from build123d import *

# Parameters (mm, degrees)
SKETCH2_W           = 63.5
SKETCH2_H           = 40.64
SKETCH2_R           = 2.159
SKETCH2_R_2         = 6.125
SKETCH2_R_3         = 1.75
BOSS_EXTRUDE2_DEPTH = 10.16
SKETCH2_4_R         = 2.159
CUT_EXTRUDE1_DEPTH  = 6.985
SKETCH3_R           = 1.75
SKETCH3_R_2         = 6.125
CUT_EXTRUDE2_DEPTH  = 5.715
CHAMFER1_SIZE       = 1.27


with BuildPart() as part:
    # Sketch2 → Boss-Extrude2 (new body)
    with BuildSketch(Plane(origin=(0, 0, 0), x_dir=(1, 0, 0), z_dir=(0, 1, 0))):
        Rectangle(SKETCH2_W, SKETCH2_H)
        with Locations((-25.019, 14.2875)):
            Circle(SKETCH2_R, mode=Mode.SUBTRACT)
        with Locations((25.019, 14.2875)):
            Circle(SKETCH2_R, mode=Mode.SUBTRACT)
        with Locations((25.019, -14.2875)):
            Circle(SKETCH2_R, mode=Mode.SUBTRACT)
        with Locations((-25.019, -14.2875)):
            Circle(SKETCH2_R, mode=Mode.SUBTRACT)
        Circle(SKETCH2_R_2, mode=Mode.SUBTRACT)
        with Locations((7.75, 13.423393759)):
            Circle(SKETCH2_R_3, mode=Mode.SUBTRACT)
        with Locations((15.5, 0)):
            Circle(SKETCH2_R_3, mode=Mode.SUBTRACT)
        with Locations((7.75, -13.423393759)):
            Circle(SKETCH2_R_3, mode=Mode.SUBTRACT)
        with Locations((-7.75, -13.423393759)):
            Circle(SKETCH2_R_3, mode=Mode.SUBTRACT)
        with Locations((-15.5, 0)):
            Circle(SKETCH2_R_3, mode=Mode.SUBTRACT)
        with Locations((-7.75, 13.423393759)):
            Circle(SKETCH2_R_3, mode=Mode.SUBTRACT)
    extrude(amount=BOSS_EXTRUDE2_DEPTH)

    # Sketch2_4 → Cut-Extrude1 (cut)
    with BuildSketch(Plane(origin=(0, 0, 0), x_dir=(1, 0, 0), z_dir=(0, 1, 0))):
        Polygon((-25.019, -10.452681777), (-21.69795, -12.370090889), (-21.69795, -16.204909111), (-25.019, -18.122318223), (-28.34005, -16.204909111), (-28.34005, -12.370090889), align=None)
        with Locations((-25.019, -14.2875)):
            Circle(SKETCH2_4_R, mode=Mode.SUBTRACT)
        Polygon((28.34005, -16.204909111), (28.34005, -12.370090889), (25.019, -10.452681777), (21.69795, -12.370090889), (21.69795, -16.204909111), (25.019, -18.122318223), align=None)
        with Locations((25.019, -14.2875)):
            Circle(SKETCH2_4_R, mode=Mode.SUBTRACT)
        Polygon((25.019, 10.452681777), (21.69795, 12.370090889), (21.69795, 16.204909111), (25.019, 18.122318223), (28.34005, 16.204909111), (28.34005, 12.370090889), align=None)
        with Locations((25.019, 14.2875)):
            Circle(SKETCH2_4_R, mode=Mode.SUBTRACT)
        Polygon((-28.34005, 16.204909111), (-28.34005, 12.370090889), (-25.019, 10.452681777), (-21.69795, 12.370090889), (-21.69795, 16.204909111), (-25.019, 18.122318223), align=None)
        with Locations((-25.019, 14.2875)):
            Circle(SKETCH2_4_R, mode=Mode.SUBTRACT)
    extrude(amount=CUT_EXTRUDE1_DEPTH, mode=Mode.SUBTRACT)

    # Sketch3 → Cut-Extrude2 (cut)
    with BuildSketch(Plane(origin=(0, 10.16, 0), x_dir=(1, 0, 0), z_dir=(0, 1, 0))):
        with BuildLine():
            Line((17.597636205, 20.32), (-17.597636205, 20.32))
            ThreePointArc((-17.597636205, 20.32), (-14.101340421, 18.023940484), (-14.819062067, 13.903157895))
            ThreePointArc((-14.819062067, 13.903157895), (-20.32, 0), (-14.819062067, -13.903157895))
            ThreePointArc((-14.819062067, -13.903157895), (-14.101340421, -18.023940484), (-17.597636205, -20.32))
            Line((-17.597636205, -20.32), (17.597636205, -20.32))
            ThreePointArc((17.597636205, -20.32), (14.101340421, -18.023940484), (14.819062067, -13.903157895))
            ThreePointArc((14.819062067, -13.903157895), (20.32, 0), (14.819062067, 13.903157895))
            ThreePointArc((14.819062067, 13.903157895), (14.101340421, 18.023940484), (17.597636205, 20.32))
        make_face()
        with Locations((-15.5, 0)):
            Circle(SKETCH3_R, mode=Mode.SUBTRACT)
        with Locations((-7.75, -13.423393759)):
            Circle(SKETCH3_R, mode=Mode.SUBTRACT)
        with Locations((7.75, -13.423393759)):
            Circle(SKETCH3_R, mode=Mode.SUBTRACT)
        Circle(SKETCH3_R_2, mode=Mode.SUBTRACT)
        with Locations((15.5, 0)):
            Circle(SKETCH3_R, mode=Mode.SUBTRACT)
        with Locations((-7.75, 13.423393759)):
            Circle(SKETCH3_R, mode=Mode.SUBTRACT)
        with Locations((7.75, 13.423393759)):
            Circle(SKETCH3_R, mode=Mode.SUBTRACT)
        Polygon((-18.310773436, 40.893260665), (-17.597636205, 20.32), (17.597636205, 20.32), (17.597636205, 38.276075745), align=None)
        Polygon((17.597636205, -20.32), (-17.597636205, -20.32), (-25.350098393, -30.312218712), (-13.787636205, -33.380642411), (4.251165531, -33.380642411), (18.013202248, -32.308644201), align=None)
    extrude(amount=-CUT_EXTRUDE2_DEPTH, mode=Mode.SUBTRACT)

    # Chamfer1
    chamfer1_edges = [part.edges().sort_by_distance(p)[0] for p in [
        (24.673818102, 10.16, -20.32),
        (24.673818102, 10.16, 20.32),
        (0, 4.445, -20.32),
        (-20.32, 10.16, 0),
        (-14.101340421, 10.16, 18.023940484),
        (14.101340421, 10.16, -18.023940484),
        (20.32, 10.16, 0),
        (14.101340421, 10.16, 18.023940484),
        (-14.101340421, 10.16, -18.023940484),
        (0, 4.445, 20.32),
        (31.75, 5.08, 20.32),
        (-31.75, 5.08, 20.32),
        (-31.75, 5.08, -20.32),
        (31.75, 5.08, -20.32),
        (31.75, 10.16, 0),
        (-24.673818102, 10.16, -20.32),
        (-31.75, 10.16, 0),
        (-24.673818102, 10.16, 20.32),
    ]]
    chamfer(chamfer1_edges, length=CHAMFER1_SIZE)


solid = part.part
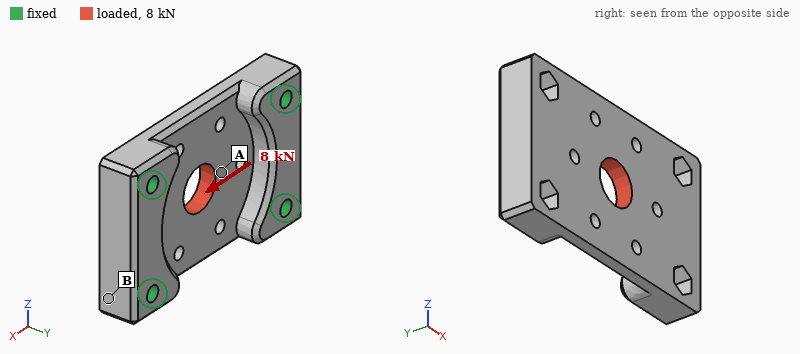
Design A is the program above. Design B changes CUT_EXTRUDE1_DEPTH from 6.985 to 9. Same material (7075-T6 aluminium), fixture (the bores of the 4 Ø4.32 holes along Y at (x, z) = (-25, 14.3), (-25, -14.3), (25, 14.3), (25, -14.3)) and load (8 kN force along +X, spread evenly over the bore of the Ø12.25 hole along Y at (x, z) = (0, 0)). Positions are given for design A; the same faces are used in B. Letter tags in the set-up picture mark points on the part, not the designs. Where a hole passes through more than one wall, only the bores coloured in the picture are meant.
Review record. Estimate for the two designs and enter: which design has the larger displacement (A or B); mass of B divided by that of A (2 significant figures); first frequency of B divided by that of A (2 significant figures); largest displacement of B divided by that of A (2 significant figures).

B
0.99
0.82
1.8
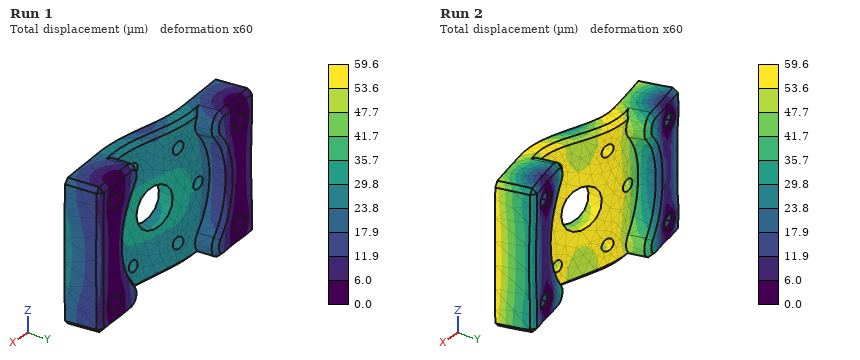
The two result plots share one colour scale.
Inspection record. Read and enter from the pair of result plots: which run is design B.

Run 2
